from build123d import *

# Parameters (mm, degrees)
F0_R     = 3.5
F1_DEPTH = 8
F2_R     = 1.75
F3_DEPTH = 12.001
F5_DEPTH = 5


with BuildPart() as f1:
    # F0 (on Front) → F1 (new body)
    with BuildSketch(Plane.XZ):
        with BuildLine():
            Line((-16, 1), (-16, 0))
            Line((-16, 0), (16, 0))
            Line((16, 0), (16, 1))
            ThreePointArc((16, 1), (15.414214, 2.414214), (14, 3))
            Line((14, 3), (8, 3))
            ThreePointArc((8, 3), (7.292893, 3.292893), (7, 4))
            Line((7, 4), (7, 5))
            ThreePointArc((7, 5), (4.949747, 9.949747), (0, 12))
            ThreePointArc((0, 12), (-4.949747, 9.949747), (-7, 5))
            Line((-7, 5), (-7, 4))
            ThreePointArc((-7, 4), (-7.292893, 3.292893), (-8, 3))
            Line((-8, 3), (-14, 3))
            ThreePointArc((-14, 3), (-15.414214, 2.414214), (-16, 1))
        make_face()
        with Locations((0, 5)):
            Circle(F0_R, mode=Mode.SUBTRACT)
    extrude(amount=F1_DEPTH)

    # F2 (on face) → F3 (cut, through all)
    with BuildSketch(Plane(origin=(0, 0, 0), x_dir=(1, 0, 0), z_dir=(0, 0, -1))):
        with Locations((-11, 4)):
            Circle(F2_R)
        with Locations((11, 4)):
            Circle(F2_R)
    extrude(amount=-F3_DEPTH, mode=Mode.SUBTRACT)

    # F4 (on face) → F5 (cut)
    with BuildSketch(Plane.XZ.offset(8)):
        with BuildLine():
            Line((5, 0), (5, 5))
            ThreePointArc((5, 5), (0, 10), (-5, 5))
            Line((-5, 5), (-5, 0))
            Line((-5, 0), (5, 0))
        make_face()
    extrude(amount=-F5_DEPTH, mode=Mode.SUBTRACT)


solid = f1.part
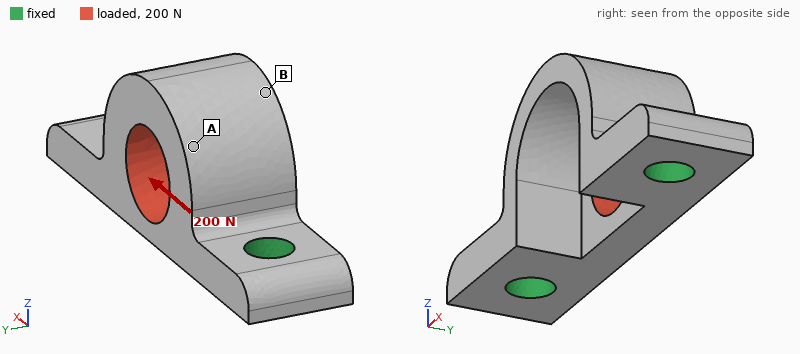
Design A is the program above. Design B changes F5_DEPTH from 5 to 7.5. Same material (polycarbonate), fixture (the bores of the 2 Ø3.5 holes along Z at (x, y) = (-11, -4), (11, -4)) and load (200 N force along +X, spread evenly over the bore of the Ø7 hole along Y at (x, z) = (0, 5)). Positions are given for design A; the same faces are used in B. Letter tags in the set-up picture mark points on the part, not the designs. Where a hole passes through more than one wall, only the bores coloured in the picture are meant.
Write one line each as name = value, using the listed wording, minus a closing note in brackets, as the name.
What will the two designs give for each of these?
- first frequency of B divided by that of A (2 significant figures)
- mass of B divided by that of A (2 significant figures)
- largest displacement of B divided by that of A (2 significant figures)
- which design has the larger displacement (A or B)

first frequency of B divided by that of A = 1.1
mass of B divided by that of A = 0.87
largest displacement of B divided by that of A = 2.6
which design has the larger displacement = B
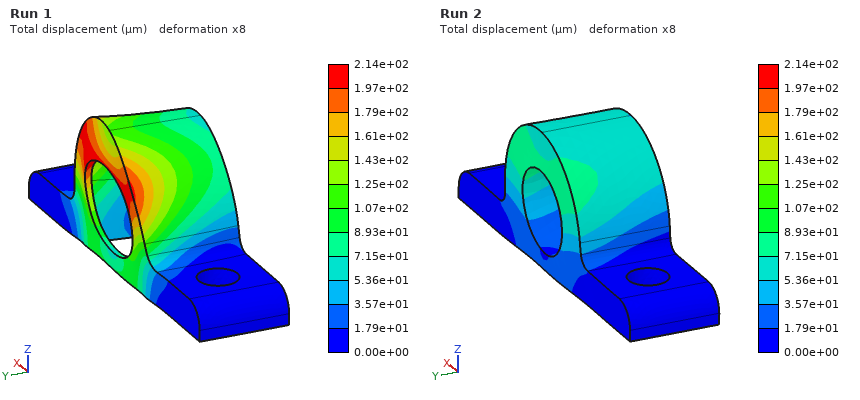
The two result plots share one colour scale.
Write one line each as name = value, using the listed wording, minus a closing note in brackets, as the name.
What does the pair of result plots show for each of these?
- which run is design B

which run is design B = Run 1
